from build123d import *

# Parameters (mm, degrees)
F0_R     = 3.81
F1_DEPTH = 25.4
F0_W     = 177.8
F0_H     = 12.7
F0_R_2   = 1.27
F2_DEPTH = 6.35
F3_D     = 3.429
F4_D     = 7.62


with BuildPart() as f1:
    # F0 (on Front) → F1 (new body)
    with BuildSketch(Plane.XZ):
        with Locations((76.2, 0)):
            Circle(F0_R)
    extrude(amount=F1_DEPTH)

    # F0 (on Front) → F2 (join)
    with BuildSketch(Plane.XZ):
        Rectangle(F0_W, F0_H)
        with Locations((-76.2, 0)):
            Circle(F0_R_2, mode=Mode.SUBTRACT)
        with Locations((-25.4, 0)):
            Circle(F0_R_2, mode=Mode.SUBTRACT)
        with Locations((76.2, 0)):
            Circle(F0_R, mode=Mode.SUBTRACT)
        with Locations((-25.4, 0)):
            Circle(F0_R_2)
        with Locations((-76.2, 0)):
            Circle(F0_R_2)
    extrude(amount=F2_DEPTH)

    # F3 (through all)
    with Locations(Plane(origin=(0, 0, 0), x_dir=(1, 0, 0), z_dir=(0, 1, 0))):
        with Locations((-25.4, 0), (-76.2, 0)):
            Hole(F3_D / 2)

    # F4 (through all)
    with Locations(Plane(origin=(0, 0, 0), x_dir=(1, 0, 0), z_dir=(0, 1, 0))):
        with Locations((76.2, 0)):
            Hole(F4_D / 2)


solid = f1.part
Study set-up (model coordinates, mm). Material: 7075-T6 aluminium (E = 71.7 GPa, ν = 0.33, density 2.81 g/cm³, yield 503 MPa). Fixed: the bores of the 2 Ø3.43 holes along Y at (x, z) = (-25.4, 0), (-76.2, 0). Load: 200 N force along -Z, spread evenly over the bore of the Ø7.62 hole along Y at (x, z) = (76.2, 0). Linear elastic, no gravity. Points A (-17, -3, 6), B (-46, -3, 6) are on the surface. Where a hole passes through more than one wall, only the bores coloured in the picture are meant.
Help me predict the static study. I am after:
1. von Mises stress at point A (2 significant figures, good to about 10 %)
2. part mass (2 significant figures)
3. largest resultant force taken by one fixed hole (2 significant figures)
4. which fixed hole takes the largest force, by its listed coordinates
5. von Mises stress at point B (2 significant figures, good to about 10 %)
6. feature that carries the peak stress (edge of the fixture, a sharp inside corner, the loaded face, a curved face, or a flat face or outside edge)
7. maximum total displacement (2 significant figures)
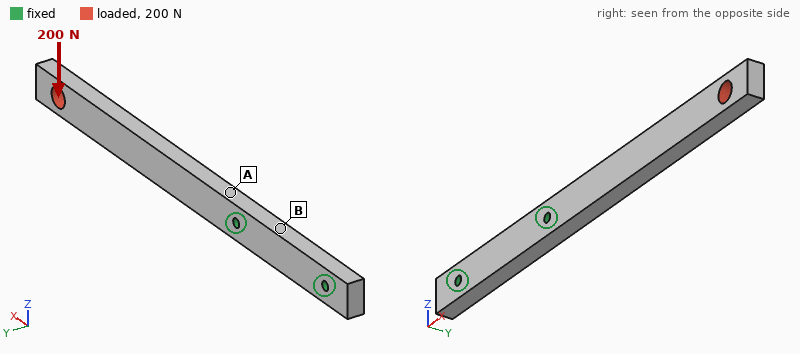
110 MPa
39 g
400 N
(-25.4, 0)
23 MPa
edge of the fixture
1.3 mm
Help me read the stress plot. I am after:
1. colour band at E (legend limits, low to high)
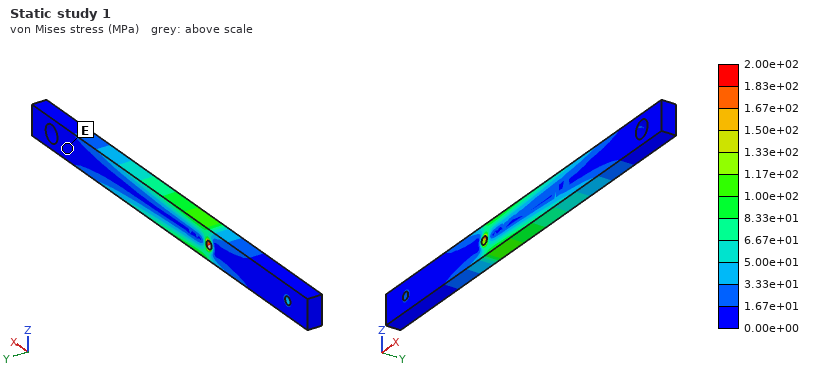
0.00e+00 to 1.67e+01 MPa
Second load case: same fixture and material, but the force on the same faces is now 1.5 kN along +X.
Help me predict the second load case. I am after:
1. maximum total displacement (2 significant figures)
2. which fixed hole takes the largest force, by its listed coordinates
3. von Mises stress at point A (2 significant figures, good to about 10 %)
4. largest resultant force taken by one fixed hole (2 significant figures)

30 µm
(-25.4, 0)
16 MPa
1.4 kN
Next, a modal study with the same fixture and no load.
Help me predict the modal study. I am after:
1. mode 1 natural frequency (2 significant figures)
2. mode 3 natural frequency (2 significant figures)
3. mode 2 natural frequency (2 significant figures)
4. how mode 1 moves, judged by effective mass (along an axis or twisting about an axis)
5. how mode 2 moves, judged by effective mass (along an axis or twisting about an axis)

410 Hz
2500 Hz
750 Hz
along Y
along Z
